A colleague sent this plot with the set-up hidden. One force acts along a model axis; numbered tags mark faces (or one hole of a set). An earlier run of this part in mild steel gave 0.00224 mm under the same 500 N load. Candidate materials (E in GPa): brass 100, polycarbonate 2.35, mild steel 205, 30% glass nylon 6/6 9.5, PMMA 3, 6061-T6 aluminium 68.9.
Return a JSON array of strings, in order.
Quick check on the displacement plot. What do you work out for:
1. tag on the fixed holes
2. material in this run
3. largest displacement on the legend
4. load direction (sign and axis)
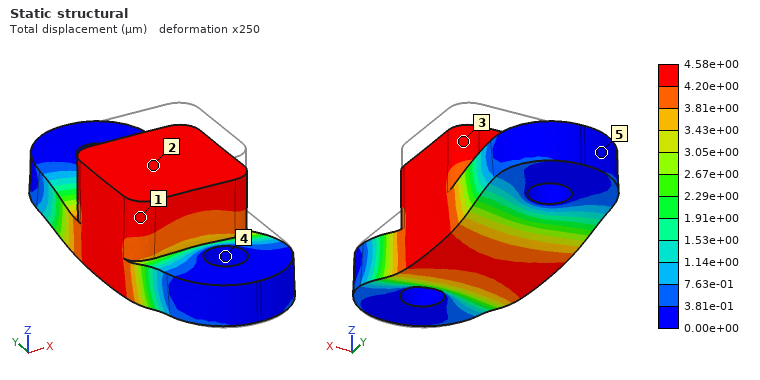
["4", "brass", "4.58e+00 µm", "-Z"]
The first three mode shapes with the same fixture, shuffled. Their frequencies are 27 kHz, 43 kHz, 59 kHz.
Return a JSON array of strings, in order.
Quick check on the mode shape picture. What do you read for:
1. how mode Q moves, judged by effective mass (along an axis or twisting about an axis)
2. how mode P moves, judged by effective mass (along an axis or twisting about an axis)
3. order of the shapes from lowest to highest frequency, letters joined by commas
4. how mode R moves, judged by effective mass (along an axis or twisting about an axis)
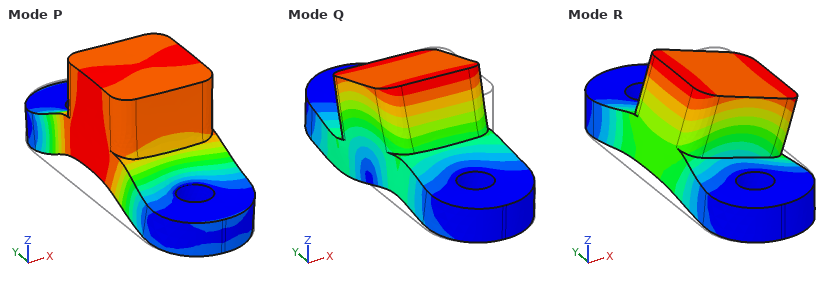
["along Y", "along Z", "R, P, Q", "along X"]
